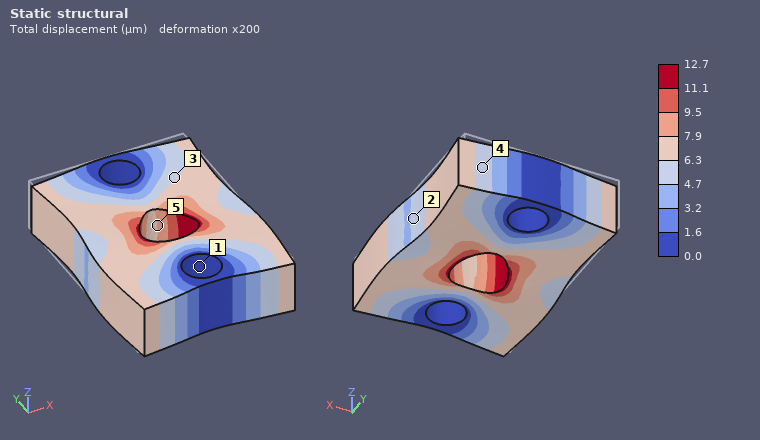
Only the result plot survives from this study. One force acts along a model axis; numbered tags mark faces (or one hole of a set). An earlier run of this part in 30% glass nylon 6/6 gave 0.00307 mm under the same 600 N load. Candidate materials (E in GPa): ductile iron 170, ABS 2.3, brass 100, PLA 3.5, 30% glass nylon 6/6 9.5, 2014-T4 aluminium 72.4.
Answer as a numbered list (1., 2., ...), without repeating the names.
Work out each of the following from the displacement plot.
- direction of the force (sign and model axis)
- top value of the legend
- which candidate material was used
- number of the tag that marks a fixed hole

1. -Y
2. 12.7 µm
3. ABS
4. 1
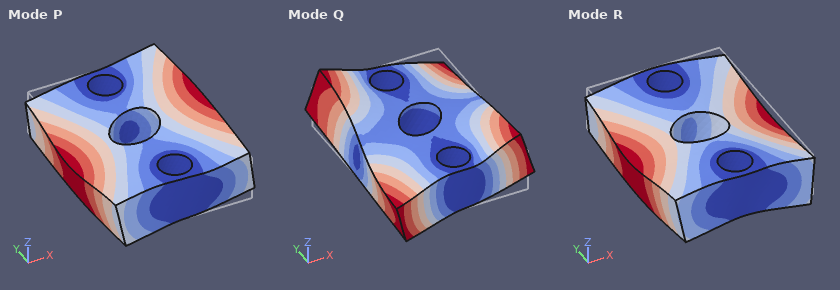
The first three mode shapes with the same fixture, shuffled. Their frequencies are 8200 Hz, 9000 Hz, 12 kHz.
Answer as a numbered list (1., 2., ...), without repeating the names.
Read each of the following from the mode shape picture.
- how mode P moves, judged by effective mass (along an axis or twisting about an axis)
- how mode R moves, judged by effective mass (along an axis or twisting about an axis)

1. twisting about Y
2. along Z
